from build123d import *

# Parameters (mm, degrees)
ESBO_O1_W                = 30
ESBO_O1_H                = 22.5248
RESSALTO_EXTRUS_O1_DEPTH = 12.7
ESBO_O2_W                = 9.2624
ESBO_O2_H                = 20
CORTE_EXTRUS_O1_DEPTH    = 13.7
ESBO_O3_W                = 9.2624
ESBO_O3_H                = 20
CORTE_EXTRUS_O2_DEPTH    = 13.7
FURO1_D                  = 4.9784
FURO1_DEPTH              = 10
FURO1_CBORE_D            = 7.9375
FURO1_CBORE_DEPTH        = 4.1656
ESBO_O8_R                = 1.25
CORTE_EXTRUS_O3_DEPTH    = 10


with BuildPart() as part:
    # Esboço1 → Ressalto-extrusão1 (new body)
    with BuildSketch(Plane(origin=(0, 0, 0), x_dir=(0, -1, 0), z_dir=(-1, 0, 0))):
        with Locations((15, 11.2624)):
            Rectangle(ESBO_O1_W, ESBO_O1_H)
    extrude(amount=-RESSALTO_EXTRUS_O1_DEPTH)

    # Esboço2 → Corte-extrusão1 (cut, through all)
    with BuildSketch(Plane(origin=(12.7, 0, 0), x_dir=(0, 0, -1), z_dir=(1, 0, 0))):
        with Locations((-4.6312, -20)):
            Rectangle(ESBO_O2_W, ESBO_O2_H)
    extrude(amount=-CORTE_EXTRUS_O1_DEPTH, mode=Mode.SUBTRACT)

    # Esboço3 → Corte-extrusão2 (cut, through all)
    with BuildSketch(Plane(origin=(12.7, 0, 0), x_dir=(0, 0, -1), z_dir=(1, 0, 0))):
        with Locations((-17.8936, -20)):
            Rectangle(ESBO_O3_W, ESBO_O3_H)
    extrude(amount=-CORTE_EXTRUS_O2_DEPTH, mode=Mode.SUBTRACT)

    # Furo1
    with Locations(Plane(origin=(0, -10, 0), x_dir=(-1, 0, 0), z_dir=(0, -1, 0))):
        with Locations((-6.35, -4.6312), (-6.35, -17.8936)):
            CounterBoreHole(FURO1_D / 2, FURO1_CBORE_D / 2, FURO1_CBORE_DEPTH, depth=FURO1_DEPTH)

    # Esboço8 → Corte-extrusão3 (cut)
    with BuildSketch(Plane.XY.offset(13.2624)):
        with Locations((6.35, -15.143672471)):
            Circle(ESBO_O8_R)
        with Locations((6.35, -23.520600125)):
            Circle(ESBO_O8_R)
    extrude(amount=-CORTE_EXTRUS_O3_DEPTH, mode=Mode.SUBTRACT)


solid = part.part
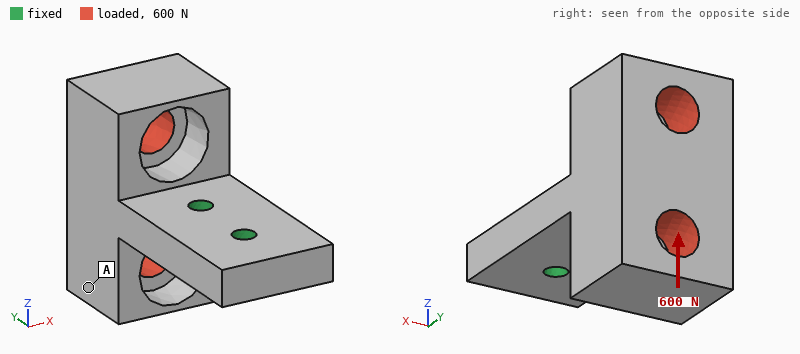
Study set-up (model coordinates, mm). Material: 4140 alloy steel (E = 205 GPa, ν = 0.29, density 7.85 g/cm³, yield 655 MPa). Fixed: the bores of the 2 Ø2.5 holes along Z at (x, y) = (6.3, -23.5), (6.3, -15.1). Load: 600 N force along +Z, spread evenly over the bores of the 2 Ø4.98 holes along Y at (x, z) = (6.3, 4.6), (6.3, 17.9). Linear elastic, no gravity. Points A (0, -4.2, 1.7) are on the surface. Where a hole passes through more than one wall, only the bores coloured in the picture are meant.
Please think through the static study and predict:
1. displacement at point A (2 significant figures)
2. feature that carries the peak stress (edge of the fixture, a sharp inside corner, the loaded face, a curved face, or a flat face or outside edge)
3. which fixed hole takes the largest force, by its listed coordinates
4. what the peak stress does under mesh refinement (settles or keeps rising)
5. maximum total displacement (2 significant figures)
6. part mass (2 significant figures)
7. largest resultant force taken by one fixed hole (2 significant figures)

35 µm
edge of the fixture
(6.3, -15.1)
keeps rising
46 µm
25 g
860 N
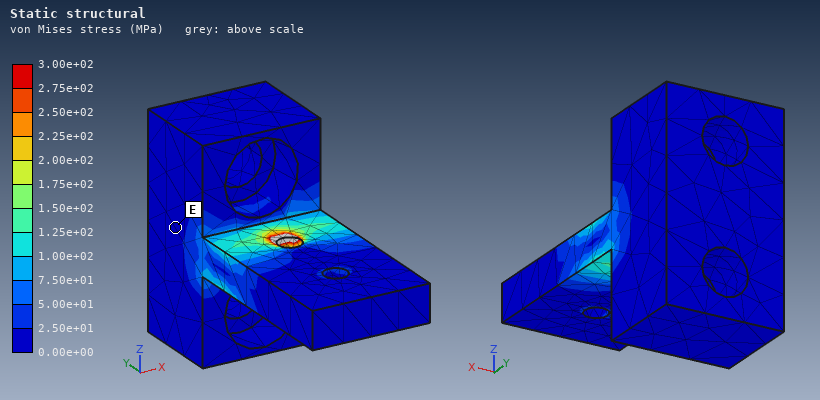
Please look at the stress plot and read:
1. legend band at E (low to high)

0.00e+00 to 2.50e+01 MPa
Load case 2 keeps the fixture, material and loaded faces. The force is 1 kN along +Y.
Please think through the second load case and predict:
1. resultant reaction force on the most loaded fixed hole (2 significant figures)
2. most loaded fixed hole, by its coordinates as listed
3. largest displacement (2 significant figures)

800 N
(6.3, -15.1)
2.2 µm
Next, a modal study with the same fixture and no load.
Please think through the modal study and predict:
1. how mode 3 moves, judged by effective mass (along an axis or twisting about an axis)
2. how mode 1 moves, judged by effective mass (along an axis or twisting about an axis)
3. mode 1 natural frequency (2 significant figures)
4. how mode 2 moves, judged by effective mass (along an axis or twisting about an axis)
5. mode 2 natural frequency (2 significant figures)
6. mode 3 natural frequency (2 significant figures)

along X
along Z
5200 Hz
twisting about Y
8900 Hz
11 kHz
